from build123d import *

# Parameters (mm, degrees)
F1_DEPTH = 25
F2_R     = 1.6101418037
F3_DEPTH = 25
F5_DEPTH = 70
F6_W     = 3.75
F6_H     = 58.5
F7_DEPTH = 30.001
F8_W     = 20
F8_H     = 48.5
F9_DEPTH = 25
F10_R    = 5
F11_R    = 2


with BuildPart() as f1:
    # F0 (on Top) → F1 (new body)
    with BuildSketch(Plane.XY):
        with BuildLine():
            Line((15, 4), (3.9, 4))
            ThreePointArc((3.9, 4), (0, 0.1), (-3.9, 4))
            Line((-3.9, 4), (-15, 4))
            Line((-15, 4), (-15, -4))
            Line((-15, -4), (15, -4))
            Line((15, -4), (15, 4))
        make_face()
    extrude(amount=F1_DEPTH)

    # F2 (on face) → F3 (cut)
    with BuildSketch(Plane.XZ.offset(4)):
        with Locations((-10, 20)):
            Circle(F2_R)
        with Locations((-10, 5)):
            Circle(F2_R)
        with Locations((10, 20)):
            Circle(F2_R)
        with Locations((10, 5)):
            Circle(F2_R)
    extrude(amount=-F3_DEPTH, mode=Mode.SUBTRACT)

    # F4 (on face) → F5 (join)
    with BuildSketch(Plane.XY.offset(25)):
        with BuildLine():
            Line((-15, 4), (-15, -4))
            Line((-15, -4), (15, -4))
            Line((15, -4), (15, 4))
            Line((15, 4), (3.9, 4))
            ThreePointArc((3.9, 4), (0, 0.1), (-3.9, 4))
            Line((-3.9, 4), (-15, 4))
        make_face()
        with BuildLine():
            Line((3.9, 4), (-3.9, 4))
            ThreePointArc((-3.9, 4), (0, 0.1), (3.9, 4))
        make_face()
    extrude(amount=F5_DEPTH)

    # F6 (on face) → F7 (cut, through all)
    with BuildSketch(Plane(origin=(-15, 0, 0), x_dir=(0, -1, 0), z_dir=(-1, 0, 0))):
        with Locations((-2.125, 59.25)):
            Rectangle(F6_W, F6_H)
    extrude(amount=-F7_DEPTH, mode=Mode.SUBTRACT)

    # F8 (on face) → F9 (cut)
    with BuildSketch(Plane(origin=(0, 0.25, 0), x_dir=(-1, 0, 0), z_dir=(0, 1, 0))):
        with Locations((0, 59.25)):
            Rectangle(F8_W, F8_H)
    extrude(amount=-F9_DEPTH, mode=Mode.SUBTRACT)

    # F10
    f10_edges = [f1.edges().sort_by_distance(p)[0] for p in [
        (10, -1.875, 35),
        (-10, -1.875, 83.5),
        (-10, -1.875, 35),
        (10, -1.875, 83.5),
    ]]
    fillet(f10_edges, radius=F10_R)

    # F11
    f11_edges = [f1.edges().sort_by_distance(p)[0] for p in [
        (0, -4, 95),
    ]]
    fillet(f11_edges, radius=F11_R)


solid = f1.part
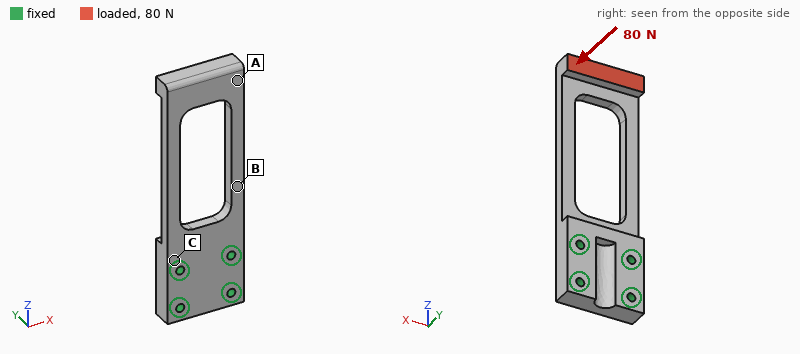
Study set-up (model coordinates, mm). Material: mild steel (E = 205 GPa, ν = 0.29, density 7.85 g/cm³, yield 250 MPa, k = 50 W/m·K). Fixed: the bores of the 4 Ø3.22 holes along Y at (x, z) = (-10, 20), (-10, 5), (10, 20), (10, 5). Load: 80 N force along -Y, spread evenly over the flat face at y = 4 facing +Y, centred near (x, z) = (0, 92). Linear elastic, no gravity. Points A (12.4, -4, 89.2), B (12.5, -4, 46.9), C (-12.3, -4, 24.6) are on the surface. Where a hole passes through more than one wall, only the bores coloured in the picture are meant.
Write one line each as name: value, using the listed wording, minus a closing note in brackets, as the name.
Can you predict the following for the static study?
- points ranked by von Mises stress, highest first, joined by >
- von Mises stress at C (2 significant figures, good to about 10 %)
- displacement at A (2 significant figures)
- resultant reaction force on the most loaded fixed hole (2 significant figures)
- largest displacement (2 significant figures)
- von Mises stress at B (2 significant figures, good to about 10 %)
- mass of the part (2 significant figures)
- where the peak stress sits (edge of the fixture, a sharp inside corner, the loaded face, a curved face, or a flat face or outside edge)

points ranked by von Mises stress, highest first, joined by >: B > C > A
von Mises stress at C: 23 MPa
displacement at A: 0.43 mm
resultant reaction force on the most loaded fixed hole: 88 N
largest displacement: 0.49 mm
von Mises stress at B: 120 MPa
mass of the part: 89 g
where the peak stress sits: a curved face
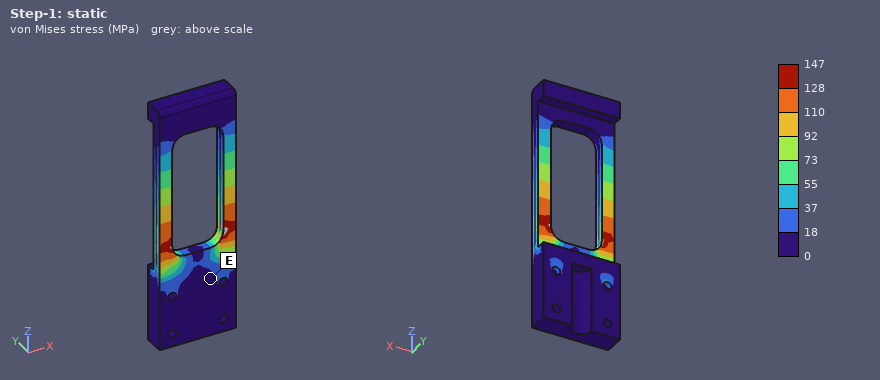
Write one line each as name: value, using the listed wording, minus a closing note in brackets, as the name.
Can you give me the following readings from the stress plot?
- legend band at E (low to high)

legend band at E: 0 to 18 MPa
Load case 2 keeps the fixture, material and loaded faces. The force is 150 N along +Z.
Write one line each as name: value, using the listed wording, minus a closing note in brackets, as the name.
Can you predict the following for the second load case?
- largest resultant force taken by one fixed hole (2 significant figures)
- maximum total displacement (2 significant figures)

largest resultant force taken by one fixed hole: 71 N
maximum total displacement: 0.13 mm
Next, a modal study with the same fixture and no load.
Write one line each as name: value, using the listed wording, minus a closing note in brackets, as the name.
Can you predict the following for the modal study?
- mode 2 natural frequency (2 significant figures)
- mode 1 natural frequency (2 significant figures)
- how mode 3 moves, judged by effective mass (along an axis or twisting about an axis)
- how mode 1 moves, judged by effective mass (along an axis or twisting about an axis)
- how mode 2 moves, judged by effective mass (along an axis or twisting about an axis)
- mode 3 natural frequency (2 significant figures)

mode 2 natural frequency: 1300 Hz
mode 1 natural frequency: 490 Hz
how mode 3 moves, judged by effective mass: twisting about Z
how mode 1 moves, judged by effective mass: along Y
how mode 2 moves, judged by effective mass: along X
mode 3 natural frequency: 1900 Hz
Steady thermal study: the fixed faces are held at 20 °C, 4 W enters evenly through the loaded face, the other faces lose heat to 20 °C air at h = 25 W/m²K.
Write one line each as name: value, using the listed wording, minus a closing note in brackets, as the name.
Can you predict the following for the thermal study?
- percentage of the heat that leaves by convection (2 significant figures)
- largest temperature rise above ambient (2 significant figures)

percentage of the heat that leaves by convection: 62 %
largest temperature rise above ambient: 55 K
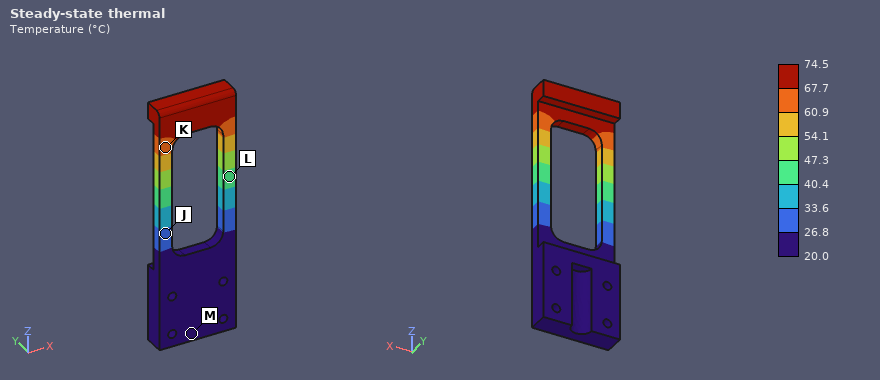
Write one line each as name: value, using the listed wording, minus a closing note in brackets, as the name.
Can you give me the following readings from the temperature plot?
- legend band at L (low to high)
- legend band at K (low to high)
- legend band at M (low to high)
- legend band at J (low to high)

legend band at L: 40.4 to 47.3 °C
legend band at K: 60.9 to 67.7 °C
legend band at M: 20.0 to 26.8 °C
legend band at J: 26.8 to 33.6 °C
